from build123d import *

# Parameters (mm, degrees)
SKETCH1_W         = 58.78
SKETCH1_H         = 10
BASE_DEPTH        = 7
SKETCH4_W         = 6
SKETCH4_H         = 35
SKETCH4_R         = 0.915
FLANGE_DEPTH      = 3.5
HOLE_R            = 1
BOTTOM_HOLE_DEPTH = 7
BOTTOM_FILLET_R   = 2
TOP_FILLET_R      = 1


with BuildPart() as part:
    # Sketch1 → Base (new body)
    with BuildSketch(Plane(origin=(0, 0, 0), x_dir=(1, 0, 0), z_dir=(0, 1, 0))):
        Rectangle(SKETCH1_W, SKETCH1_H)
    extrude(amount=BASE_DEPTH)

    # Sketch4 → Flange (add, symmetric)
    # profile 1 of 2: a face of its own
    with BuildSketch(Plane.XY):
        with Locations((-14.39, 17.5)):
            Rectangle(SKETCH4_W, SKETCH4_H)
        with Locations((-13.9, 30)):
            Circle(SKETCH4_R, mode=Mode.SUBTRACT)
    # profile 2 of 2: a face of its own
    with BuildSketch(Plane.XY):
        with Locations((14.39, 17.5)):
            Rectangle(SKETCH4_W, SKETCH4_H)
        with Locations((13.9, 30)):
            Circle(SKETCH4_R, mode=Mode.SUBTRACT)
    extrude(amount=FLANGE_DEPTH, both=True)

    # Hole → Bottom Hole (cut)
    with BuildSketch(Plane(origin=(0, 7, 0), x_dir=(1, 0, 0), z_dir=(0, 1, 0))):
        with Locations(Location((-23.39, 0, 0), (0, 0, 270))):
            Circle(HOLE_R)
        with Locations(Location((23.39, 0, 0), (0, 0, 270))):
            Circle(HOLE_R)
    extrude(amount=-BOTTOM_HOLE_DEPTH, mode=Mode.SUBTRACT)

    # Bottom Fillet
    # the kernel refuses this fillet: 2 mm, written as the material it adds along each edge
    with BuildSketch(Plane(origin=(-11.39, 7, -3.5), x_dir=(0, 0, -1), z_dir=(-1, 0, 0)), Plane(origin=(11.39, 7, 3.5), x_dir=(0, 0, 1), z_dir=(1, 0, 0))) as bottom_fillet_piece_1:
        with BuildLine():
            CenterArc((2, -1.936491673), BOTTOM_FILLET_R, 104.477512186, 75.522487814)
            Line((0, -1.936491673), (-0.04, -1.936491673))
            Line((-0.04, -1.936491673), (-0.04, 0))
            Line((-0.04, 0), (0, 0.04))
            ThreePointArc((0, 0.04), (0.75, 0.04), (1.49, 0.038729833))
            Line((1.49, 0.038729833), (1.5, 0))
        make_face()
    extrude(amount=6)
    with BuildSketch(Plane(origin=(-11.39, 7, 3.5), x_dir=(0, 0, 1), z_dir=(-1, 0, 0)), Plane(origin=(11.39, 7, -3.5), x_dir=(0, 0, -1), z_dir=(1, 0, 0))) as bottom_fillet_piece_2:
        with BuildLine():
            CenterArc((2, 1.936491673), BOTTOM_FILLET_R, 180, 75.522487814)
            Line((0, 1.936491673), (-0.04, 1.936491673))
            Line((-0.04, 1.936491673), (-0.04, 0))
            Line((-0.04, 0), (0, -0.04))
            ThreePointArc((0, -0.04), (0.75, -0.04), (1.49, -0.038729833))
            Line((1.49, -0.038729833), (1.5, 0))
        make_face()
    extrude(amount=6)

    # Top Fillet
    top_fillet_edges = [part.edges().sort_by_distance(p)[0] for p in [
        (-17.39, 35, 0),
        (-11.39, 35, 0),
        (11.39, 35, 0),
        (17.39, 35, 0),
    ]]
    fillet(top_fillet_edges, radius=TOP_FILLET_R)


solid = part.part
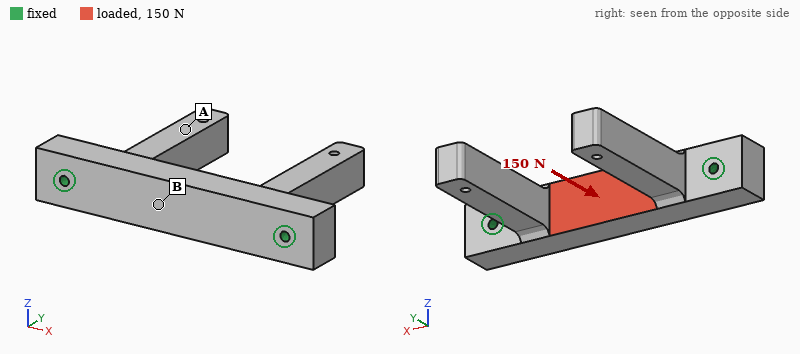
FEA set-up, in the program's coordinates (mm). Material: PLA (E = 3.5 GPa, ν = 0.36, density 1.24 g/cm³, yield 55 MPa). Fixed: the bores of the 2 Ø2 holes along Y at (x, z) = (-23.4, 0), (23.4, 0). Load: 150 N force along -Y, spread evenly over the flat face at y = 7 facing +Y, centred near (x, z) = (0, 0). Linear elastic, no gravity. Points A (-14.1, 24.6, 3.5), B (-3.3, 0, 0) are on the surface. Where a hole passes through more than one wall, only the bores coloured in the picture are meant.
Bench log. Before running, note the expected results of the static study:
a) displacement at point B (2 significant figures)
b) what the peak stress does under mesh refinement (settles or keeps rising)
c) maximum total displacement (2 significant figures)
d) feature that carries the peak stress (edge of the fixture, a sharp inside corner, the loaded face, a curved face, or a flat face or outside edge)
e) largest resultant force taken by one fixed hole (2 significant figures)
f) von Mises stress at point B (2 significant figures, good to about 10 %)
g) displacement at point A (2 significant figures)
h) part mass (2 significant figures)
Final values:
0.085 mm
keeps rising
0.17 mm
edge of the fixture
75 N
6.2 MPa
0.12 mm
7.9 g
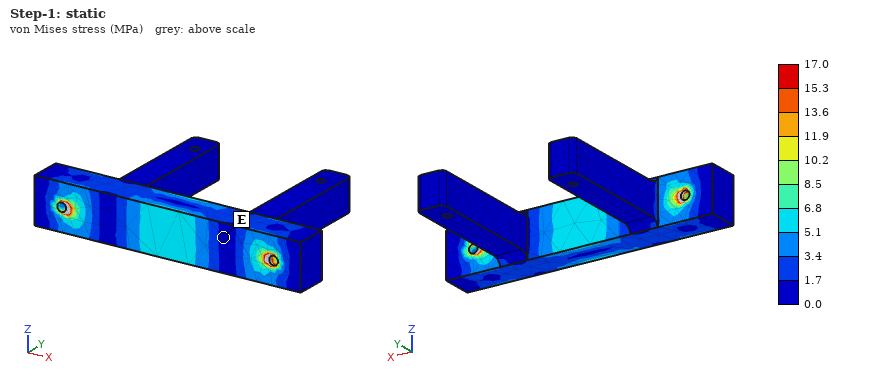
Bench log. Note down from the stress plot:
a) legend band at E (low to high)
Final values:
0.0 to 1.7 MPa
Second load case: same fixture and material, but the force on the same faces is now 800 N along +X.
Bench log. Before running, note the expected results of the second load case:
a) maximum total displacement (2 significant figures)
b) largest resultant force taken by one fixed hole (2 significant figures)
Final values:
45 µm
410 N
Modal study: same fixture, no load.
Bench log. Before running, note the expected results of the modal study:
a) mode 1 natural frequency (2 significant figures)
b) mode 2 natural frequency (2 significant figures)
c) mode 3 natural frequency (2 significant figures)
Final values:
1600 Hz
1600 Hz
1800 Hz
